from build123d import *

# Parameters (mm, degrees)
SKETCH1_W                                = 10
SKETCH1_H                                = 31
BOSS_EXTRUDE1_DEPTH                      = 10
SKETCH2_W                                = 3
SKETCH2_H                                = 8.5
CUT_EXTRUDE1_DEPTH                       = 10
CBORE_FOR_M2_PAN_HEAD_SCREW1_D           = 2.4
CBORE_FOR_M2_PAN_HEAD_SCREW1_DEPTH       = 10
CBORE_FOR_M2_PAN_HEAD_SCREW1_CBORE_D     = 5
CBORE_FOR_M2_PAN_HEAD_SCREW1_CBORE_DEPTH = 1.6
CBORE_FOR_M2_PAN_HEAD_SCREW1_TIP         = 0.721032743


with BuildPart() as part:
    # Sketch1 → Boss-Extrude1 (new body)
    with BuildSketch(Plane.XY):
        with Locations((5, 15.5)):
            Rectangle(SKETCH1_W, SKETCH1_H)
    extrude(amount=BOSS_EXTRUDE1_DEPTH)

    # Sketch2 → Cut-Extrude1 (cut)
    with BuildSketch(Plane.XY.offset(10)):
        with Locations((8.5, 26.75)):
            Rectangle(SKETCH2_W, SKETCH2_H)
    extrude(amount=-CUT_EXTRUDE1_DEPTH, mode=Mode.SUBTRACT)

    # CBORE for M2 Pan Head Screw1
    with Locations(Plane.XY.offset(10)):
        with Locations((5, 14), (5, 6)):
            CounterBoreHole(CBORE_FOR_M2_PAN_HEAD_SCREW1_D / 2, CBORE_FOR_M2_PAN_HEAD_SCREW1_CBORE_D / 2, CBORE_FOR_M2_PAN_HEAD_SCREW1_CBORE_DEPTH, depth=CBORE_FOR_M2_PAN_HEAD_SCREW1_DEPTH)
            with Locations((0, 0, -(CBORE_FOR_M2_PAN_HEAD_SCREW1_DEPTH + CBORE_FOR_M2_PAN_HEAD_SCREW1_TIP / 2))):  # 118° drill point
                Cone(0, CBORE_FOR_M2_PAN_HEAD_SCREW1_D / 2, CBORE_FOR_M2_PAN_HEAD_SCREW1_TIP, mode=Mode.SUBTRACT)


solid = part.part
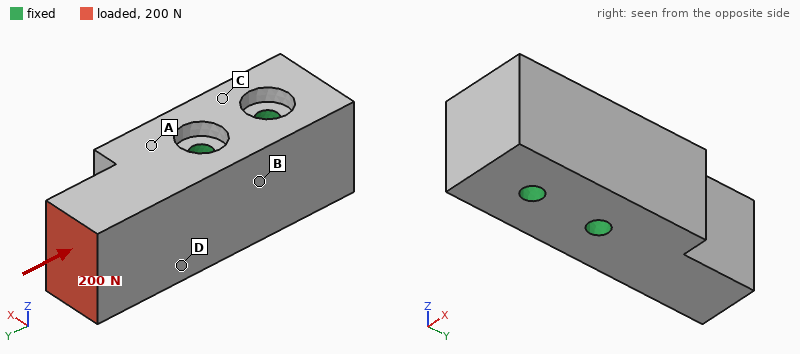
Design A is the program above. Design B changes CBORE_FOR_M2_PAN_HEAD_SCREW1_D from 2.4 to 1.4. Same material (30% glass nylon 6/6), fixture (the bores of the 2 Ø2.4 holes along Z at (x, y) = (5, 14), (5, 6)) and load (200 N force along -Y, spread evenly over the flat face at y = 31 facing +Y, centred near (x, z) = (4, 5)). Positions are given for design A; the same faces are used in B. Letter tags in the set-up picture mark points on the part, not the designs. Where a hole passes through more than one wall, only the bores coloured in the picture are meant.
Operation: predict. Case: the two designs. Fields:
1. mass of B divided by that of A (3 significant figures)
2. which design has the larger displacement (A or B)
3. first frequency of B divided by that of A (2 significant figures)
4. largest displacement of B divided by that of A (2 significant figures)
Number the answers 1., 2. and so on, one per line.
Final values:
1. 1.02
2. B
3. 0.91
4. 1.1
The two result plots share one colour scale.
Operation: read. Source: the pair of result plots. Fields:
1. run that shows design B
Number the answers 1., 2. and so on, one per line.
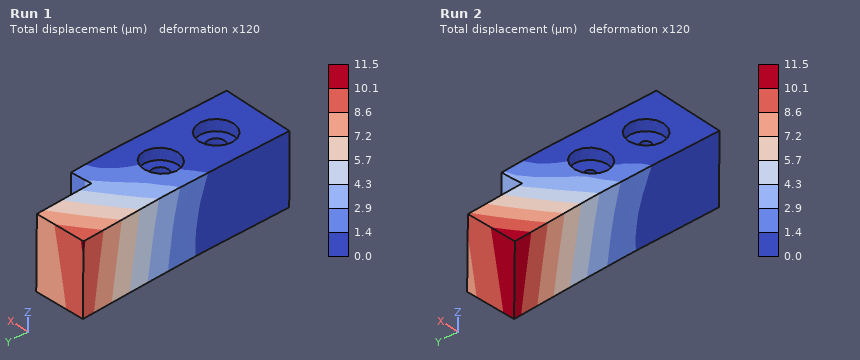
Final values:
1. Run 2
